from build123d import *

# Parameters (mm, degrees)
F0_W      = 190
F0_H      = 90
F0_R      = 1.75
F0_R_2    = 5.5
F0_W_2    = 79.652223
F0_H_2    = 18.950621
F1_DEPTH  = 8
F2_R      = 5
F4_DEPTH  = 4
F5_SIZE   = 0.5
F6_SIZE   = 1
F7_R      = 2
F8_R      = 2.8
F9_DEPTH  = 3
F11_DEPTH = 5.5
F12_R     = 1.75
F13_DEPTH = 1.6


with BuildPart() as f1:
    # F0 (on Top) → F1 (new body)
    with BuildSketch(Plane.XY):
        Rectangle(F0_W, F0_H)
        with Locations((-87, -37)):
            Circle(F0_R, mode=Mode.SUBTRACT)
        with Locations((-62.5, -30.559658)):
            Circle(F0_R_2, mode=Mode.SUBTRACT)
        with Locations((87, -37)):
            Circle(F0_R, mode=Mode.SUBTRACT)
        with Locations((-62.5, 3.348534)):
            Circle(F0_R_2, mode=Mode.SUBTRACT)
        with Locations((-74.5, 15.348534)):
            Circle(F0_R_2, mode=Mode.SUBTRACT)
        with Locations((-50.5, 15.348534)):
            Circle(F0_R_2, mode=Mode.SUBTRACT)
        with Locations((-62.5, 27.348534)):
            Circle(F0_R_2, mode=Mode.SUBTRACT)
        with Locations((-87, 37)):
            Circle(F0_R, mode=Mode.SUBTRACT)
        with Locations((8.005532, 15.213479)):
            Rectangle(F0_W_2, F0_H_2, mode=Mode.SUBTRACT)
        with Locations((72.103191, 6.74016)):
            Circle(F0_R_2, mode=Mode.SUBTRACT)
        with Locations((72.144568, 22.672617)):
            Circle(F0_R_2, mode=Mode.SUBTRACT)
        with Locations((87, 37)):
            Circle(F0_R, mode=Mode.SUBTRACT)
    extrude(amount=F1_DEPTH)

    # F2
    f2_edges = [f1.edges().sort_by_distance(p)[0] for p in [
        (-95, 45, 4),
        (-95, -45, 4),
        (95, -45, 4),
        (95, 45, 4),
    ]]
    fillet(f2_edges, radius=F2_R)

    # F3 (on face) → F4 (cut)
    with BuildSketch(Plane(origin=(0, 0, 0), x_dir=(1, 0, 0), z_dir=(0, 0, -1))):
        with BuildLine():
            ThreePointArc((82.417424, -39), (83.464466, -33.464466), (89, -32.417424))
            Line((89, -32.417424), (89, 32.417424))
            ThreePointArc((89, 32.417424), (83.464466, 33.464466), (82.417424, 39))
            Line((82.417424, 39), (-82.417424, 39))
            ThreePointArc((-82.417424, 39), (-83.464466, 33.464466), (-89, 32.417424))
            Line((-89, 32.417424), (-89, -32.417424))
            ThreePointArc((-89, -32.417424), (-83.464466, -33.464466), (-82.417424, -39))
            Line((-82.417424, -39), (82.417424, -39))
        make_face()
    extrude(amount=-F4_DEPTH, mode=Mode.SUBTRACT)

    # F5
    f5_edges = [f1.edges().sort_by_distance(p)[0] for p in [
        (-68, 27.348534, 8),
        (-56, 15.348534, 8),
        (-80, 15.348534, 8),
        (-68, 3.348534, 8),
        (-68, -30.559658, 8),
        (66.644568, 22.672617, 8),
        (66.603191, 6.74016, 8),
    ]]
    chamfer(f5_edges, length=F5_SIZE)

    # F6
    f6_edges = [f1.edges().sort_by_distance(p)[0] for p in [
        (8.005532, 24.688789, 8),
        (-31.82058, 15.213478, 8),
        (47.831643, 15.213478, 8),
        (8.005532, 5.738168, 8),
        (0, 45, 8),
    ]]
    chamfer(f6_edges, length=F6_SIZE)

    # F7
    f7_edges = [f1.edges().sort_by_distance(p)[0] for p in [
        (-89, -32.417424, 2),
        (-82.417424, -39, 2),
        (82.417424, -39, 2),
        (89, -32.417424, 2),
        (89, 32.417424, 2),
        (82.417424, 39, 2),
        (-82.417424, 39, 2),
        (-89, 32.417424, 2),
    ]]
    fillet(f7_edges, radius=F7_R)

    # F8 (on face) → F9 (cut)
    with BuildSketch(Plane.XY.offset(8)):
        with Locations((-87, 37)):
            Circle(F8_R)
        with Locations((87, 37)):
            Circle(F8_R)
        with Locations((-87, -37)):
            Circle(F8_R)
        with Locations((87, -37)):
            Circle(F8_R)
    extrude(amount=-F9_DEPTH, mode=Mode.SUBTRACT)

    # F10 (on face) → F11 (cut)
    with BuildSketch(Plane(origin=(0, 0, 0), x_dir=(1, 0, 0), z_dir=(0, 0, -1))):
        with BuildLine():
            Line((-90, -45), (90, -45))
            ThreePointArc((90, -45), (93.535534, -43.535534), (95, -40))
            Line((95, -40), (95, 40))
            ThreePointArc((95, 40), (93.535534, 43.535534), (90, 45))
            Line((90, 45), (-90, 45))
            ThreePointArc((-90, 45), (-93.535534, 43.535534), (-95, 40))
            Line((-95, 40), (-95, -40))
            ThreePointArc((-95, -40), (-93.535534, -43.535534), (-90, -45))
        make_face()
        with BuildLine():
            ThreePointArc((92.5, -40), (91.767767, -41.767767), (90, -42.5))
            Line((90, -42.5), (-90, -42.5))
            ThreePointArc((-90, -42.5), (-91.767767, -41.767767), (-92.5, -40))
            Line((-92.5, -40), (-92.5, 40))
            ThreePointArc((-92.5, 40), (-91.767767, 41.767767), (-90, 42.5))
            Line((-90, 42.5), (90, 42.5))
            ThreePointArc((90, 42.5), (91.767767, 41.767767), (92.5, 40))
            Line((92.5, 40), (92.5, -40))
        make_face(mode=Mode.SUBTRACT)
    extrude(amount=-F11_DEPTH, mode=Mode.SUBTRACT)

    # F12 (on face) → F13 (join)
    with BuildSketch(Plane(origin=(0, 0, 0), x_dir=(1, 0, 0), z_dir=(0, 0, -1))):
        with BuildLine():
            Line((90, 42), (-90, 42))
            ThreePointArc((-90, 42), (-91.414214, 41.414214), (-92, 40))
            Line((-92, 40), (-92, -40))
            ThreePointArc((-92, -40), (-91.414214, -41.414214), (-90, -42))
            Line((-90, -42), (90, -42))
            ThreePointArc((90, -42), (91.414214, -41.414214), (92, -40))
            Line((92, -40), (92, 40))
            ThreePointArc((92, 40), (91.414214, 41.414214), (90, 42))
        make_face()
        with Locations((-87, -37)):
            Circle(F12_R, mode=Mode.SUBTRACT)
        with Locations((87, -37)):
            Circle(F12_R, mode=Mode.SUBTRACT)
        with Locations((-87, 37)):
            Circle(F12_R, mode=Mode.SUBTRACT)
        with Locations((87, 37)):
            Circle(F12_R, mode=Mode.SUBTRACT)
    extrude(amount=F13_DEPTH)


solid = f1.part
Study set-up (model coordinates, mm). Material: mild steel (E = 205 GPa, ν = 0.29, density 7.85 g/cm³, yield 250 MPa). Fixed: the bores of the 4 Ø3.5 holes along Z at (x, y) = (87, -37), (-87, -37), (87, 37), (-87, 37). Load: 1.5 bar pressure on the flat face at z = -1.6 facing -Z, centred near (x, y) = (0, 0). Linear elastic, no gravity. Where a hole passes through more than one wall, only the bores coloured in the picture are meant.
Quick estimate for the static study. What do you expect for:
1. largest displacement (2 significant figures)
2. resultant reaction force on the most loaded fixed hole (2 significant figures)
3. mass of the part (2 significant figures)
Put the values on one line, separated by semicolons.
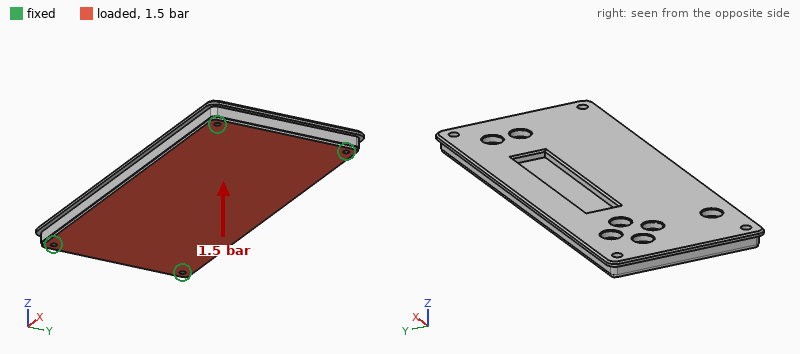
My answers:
0.29 mm; 720 N; 700 g
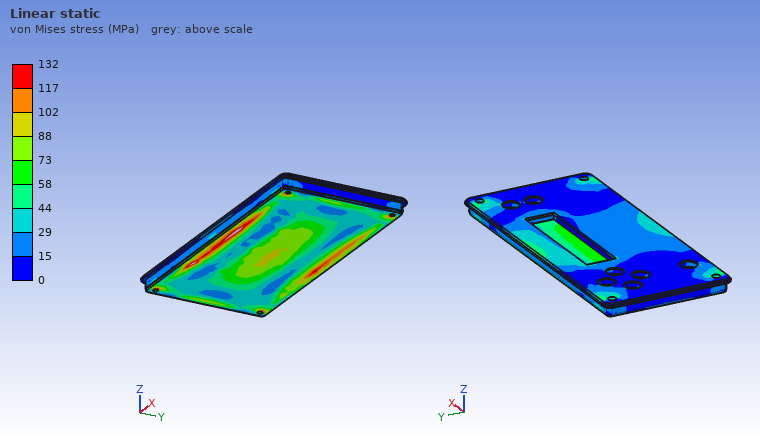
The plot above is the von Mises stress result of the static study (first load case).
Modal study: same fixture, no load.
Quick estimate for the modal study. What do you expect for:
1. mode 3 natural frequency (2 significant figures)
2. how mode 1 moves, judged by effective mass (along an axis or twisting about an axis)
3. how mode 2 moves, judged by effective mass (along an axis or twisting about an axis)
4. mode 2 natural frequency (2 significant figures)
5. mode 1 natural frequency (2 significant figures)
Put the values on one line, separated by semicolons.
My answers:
1800 Hz; along Z; twisting about X; 1600 Hz; 1000 Hz
